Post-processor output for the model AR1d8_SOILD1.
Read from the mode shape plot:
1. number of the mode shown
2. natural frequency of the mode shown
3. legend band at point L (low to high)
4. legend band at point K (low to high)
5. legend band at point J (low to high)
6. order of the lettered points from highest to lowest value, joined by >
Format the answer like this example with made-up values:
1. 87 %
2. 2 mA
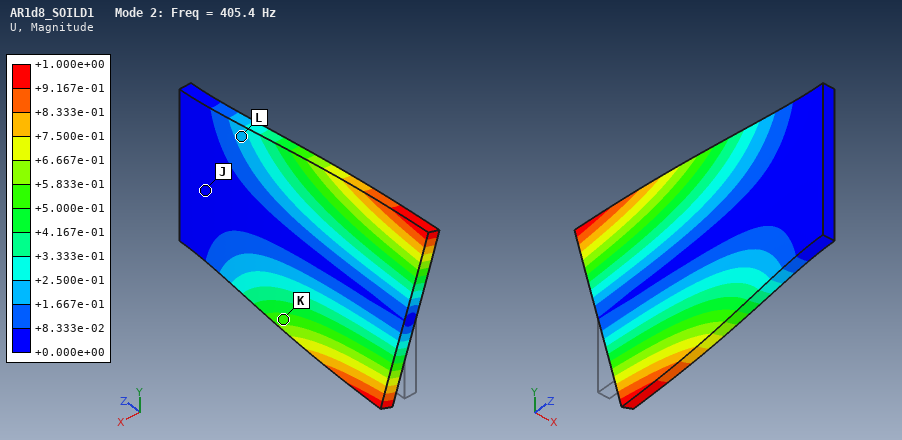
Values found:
1. 2
2. 405.4 Hz
3. +1.667e-01 to +2.500e-01
4. +5.000e-01 to +5.833e-01
5. +0.000e+00 to +8.333e-02
6. K > L > J
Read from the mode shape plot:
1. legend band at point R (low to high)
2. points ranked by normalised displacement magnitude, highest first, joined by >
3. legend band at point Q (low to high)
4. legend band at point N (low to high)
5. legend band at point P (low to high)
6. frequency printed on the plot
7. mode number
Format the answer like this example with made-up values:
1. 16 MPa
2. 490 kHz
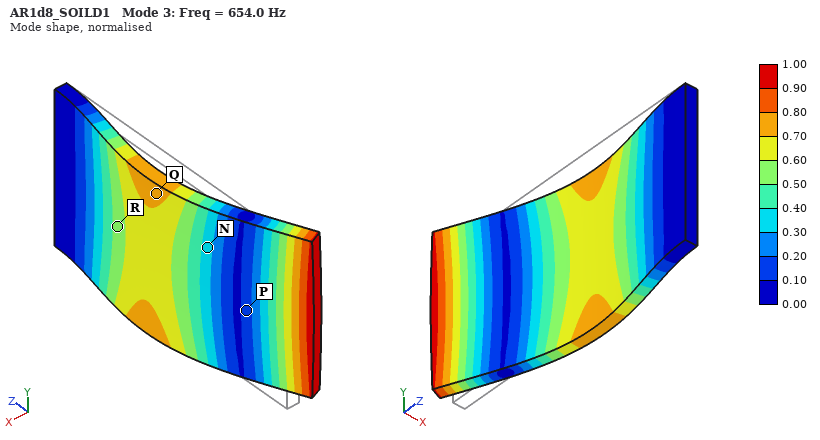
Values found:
1. 0.50 to 0.60
2. Q > R > N > P
3. 0.70 to 0.80
4. 0.30 to 0.40
5. 0.10 to 0.20
6. 654.0 Hz
7. 3
